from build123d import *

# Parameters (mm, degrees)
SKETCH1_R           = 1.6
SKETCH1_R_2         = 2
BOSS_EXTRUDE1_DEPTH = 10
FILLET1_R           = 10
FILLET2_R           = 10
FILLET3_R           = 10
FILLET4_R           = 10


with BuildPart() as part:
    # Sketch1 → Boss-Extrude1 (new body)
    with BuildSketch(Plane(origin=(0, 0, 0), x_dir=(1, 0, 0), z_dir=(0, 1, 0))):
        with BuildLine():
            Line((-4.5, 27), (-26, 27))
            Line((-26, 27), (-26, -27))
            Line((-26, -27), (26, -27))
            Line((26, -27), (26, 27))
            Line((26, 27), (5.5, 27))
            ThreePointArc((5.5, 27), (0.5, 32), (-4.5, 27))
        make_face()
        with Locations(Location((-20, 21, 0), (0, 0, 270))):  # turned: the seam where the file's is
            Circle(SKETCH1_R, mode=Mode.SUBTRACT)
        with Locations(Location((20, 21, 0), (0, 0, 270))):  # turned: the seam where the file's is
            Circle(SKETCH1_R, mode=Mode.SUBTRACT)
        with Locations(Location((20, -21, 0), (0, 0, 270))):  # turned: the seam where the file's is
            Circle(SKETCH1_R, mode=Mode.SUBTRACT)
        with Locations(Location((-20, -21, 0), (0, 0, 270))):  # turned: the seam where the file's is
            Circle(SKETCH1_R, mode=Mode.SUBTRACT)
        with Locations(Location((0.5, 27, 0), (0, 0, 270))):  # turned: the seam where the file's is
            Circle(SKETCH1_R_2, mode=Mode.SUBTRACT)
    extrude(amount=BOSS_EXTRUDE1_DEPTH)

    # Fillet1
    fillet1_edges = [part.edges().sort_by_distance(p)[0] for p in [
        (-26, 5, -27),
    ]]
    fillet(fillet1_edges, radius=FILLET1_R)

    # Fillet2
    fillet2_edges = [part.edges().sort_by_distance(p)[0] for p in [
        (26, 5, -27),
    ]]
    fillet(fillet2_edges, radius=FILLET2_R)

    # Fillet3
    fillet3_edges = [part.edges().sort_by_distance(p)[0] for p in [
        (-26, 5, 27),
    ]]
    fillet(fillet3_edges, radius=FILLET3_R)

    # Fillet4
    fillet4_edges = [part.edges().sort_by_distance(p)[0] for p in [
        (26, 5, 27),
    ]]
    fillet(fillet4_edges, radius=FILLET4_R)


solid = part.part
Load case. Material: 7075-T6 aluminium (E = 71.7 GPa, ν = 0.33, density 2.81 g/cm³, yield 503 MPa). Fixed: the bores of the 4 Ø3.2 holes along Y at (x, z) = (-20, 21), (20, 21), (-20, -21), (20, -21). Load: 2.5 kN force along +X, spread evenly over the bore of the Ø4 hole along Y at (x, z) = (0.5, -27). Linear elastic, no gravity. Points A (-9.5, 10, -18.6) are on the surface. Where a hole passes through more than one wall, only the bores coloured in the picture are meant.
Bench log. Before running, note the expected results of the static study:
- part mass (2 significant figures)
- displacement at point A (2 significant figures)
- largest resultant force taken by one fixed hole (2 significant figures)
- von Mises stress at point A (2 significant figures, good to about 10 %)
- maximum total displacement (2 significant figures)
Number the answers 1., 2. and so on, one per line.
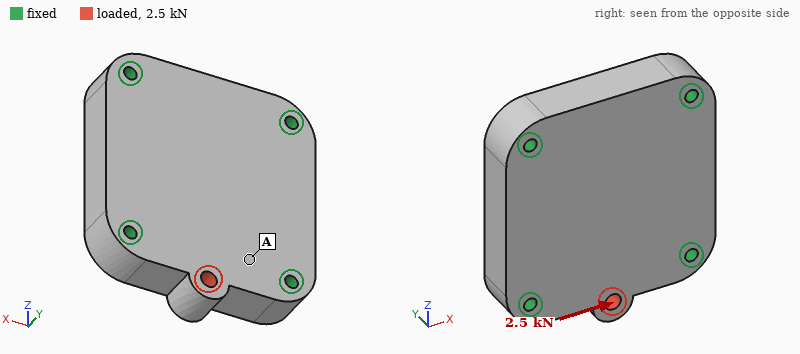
1. 76 g
2. 1.6 µm
3. 1.3 kN
4. 7.2 MPa
5. 8.1 µm
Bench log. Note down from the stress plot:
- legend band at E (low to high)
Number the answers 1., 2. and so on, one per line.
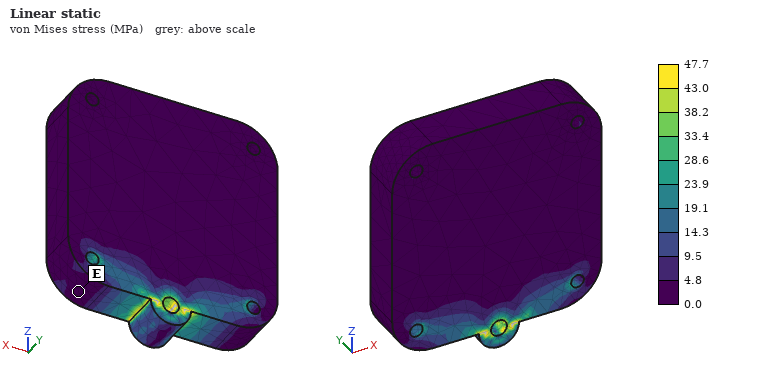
1. 0.0 to 4.8 MPa
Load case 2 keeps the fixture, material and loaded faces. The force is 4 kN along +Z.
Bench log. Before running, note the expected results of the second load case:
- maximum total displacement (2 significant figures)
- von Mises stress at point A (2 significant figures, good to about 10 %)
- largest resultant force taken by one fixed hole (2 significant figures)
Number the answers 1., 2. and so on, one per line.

1. 11 µm
2. 14 MPa
3. 1.2 kN
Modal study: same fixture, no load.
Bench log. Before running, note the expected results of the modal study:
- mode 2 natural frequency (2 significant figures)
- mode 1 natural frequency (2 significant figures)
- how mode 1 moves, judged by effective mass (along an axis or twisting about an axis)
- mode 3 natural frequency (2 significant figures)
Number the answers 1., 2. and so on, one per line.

1. 22 kHz
2. 15 kHz
3. along Y
4. 23 kHz
